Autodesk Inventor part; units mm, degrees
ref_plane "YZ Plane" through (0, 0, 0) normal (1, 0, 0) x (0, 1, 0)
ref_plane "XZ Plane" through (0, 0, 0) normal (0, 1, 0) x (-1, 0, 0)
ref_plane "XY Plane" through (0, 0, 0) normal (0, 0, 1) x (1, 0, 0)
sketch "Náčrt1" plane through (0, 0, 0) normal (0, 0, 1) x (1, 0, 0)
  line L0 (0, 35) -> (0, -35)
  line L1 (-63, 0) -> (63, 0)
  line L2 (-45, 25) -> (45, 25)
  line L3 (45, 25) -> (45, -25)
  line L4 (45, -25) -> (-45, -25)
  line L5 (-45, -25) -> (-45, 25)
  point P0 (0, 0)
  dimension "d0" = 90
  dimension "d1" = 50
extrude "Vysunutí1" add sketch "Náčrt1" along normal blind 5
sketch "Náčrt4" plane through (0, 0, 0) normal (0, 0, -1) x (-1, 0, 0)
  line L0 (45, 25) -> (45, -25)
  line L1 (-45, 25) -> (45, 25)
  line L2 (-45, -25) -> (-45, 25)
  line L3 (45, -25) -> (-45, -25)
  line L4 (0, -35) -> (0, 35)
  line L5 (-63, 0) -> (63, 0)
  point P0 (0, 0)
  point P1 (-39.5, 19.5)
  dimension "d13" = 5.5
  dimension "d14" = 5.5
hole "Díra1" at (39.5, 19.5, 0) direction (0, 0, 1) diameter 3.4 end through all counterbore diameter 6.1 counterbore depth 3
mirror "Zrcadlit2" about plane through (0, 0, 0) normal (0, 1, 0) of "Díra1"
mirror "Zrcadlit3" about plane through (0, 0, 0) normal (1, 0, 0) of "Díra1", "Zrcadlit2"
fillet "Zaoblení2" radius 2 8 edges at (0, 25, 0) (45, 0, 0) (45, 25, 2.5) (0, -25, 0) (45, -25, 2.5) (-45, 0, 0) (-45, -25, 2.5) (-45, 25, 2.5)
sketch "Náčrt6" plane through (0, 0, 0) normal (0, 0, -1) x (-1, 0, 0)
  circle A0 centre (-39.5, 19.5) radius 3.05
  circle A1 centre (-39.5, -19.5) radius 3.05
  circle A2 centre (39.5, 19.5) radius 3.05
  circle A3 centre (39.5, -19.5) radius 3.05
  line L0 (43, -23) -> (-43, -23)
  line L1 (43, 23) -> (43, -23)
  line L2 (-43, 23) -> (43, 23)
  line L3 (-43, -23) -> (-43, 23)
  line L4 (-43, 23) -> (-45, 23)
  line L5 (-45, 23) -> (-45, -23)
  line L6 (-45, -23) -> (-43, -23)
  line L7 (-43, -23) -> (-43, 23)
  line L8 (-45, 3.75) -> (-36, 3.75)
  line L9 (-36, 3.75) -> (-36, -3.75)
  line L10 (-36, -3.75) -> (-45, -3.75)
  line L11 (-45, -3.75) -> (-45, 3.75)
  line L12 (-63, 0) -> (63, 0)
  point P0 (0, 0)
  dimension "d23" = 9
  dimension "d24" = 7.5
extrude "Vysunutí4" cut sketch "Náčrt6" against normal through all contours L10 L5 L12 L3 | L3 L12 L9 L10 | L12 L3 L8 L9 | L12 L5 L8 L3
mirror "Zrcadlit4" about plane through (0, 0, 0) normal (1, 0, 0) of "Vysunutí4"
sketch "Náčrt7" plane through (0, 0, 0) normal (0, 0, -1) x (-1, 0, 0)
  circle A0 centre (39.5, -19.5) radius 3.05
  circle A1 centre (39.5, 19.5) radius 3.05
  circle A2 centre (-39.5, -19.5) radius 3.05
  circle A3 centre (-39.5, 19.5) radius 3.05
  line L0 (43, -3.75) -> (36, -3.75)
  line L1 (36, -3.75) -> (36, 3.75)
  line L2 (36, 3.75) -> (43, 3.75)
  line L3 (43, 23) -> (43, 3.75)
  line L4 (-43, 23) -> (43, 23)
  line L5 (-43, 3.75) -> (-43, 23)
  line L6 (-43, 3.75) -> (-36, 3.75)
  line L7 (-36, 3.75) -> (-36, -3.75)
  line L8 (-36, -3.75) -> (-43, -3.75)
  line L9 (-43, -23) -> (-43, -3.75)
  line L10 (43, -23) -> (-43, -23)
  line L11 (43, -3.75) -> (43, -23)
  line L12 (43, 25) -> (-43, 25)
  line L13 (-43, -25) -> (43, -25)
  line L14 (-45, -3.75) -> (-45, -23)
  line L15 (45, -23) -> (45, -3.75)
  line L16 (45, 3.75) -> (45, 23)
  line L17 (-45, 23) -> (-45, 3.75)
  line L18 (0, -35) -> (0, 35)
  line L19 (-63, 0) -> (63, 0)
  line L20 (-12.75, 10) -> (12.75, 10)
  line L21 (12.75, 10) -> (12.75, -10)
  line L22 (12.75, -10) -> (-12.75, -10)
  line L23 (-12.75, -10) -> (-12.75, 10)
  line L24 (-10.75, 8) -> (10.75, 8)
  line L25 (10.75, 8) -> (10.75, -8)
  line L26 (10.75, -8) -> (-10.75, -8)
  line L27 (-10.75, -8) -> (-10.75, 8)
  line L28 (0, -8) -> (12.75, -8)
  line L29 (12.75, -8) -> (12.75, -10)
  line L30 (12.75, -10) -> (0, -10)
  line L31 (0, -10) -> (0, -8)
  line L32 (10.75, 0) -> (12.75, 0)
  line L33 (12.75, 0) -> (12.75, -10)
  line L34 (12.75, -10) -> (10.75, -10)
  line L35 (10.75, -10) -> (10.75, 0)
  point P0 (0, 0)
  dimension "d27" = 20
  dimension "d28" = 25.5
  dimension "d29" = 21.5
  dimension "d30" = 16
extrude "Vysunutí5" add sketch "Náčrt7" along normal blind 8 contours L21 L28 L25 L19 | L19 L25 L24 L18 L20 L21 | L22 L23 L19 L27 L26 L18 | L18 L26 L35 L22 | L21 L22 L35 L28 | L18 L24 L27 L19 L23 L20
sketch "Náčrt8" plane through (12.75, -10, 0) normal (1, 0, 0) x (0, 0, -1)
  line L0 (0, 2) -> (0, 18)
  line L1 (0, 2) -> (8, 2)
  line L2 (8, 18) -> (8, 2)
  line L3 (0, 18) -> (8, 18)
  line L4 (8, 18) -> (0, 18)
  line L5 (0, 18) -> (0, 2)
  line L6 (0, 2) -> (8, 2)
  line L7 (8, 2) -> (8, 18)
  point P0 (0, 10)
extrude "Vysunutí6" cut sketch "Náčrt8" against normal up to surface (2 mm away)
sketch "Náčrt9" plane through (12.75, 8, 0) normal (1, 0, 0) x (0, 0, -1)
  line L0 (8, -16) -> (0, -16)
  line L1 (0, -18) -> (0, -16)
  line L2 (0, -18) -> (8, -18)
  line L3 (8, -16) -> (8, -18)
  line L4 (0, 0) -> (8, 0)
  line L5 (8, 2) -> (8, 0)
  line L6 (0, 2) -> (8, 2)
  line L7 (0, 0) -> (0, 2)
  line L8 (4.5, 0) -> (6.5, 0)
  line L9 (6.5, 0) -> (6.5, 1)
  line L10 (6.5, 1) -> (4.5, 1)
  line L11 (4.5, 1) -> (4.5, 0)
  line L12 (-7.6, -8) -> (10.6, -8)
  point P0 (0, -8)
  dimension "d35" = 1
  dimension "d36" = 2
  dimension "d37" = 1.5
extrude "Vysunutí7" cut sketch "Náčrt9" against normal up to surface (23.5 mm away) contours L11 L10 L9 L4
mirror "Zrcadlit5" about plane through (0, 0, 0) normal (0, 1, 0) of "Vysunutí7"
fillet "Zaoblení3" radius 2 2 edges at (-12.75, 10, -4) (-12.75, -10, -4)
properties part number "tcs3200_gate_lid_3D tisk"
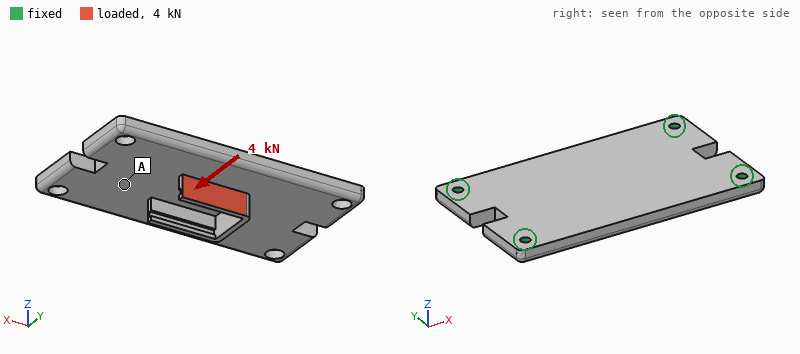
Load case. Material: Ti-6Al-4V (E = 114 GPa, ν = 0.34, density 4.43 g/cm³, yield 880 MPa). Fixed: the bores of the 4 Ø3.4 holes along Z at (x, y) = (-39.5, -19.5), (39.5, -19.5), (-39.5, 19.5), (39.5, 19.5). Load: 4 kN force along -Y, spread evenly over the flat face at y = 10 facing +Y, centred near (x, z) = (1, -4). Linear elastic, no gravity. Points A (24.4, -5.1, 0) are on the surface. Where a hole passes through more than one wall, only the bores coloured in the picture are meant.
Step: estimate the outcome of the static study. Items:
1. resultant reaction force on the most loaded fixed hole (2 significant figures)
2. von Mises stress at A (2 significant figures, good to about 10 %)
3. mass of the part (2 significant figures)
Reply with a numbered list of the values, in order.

1. 1.6 kN
2. 53 MPa
3. 98 g
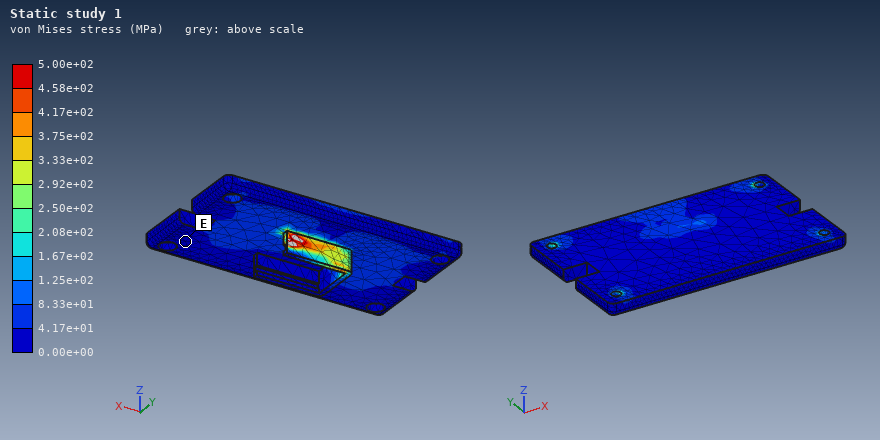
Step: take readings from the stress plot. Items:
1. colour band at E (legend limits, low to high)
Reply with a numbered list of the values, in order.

1. 0.00e+00 to 4.17e+01 MPa
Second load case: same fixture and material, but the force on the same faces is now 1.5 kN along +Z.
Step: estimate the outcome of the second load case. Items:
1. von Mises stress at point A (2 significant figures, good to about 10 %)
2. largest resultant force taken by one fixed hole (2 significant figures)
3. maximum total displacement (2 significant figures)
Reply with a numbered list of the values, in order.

1. 25 MPa
2. 1.3 kN
3. 0.13 mm
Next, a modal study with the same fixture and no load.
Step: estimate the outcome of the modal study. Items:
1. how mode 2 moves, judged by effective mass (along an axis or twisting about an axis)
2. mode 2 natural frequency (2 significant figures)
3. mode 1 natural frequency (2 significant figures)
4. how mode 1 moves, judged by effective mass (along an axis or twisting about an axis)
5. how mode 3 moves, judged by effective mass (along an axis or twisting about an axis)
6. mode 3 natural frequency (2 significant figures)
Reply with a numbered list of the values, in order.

1. twisting about X
2. 4900 Hz
3. 3000 Hz
4. along Z
5. twisting about Y
6. 7700 Hz
